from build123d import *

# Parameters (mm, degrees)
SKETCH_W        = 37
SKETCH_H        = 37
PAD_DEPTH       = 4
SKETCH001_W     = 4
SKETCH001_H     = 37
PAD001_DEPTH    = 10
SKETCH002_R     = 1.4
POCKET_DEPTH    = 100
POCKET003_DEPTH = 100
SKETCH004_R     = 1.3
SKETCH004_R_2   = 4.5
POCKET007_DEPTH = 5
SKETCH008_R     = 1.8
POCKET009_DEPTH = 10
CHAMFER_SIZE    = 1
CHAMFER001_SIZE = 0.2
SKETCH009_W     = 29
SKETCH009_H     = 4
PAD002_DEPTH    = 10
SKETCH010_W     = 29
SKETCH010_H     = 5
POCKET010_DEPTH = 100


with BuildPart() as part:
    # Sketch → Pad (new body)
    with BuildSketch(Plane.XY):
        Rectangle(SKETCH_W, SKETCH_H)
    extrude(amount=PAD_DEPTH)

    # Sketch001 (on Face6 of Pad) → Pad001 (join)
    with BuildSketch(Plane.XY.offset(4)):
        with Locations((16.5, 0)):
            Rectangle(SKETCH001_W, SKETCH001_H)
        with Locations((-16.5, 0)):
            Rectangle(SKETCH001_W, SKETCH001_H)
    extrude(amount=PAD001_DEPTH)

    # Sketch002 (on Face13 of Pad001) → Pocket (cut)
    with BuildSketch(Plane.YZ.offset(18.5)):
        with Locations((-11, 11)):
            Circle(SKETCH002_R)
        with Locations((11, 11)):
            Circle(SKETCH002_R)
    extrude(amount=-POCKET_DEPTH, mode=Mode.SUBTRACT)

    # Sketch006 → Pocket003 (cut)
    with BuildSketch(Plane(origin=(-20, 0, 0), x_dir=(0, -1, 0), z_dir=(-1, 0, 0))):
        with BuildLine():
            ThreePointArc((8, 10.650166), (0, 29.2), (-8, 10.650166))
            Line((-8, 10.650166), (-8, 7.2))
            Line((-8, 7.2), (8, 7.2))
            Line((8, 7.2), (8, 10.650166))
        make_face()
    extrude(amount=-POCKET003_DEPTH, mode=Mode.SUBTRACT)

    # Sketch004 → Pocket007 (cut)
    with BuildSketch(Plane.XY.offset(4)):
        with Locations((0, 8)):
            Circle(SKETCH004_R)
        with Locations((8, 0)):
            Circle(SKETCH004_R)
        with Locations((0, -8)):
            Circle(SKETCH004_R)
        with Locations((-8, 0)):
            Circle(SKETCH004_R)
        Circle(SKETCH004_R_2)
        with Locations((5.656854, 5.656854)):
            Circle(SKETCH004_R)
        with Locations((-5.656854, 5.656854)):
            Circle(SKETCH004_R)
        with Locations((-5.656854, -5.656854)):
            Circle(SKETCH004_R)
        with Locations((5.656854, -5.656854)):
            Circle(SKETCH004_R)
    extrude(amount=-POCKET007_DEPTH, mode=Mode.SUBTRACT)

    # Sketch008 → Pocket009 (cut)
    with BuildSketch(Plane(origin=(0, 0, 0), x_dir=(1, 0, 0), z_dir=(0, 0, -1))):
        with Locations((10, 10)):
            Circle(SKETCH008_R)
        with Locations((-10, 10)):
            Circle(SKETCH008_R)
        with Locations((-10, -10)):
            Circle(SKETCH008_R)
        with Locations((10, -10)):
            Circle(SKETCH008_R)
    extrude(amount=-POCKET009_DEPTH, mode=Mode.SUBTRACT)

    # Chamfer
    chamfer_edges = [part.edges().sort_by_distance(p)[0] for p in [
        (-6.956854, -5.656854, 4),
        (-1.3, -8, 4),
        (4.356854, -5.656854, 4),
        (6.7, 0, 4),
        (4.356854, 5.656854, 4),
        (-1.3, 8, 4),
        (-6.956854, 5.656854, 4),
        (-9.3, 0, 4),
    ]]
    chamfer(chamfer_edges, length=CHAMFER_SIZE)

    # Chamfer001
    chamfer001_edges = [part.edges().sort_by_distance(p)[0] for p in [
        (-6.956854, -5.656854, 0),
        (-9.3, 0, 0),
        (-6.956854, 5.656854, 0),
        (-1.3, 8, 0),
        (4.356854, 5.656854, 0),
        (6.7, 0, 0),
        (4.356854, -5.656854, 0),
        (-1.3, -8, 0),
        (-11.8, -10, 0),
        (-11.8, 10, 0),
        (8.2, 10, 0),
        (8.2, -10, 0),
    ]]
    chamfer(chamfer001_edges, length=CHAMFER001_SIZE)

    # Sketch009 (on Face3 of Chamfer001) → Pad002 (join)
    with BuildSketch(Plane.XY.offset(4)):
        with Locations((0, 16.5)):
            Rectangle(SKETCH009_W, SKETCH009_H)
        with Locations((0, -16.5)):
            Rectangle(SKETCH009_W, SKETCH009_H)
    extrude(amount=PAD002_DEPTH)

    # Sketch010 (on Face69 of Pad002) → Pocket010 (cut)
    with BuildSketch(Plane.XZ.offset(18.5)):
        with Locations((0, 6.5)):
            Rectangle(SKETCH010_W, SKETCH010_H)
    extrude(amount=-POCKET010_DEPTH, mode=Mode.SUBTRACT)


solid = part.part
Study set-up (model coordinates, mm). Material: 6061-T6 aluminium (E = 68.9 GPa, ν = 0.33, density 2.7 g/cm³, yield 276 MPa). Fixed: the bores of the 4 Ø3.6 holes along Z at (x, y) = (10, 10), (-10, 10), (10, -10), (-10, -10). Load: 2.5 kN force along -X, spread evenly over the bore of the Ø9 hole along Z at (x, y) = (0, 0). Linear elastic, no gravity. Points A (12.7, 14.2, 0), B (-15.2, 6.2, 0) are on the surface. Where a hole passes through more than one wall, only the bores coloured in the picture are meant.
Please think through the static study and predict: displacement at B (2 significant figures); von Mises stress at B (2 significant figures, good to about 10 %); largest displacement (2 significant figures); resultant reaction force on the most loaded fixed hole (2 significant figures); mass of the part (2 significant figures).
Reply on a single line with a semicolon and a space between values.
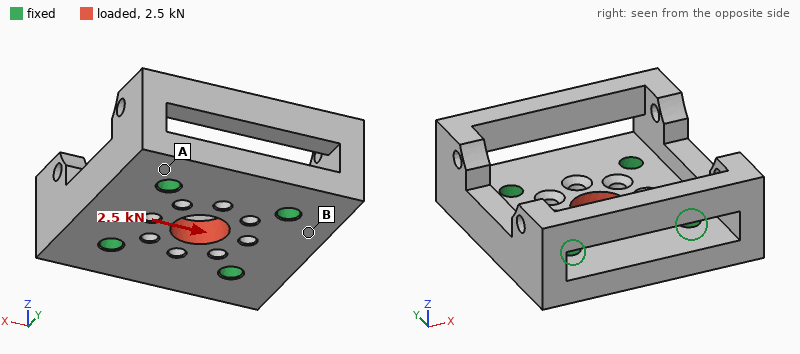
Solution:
1.4 µm; 11 MPa; 5.2 µm; 650 N; 21 g
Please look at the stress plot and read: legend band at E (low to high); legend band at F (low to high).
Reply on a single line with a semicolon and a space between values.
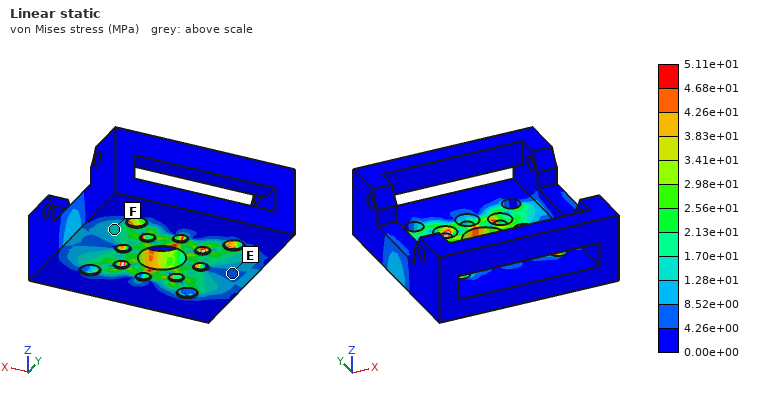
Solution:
4.26e+00 to 8.52e+00 MPa; 1.28e+01 to 1.70e+01 MPa
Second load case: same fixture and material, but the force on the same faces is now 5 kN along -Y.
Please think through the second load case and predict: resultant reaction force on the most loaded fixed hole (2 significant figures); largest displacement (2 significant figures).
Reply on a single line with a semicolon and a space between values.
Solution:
1.3 kN; 10 µm
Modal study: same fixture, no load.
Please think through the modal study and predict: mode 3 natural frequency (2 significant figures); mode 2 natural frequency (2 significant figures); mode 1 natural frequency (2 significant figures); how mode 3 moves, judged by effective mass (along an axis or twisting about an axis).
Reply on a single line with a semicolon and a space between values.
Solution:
13 kHz; 12 kHz; 12 kHz; along X
